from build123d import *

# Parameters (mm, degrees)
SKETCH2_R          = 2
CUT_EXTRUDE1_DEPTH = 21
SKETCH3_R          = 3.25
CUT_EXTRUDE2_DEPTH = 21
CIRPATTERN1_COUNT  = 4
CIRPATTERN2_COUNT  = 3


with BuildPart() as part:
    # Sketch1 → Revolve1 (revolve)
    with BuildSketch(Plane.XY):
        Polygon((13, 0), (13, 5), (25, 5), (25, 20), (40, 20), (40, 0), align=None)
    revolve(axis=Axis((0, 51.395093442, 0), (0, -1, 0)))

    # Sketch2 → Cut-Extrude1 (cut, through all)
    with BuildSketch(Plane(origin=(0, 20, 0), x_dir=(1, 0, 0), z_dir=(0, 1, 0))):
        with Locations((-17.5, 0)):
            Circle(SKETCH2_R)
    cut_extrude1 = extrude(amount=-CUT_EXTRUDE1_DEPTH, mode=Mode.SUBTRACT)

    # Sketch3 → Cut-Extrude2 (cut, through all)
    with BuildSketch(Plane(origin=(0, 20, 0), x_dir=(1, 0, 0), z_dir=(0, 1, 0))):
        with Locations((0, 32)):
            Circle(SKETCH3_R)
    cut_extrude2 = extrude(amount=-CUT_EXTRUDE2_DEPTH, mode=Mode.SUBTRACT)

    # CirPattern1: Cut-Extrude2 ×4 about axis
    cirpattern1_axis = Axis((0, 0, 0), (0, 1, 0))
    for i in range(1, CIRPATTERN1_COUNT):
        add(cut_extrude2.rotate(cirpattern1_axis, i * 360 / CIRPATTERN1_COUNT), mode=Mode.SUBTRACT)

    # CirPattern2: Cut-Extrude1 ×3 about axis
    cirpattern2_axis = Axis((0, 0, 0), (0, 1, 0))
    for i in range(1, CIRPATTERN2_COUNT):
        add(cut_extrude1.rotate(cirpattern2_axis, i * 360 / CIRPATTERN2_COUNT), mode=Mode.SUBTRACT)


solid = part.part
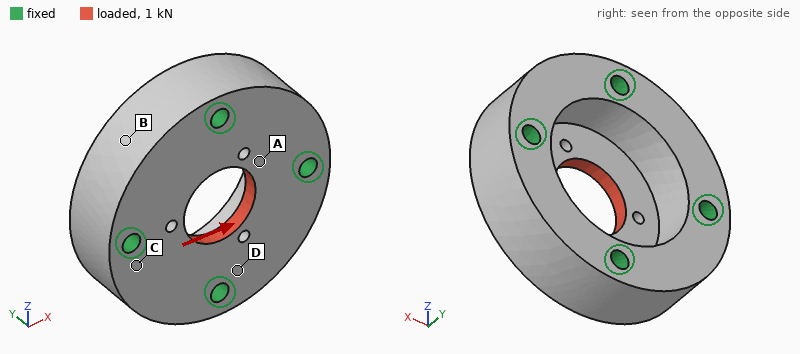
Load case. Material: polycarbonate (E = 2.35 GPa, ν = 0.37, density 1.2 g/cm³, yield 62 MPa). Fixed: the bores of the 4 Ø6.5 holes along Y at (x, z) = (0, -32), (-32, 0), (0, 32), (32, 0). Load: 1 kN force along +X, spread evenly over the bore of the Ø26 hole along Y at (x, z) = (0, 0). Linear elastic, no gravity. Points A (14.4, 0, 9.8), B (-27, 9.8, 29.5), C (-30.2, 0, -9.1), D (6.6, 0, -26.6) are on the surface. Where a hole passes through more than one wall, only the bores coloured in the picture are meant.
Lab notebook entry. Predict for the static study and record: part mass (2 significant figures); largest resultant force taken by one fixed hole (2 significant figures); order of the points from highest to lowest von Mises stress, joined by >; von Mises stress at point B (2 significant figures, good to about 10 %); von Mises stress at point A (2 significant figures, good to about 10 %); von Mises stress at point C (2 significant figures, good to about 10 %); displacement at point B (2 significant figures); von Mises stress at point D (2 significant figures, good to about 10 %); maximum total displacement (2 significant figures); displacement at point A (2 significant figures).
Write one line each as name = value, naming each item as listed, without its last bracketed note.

part mass = 79 g
largest resultant force taken by one fixed hole = 280 N
order of the points from highest to lowest von Mises stress, joined by > = A > C > D > B
von Mises stress at point B = 0.49 MPa
von Mises stress at point A = 2.4 MPa
von Mises stress at point C = 1.5 MPa
displacement at point B = 8.4 µm
von Mises stress at point D = 1.0 MPa
maximum total displacement = 33 µm
displacement at point A = 22 µm
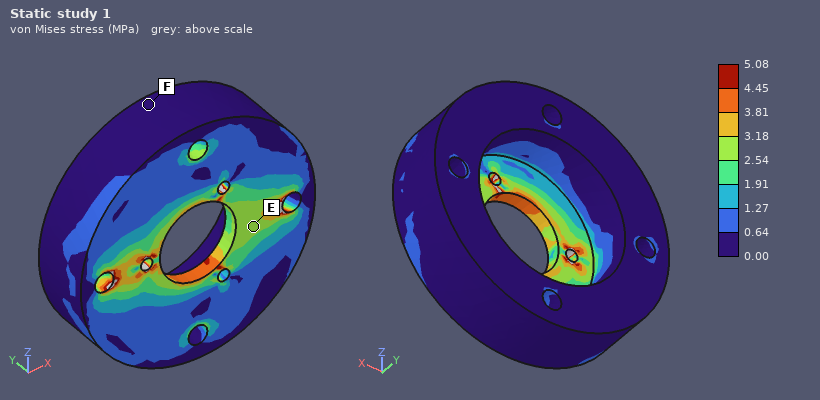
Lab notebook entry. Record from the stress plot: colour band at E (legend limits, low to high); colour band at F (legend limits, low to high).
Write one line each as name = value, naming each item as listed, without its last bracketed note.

colour band at E = 2.54 to 3.18 MPa
colour band at F = 0.00 to 0.64 MPa
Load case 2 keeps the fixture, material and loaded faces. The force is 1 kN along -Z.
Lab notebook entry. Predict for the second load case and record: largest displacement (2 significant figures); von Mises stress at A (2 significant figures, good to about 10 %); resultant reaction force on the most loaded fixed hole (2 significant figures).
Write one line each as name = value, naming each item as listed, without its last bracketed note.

largest displacement = 33 µm
von Mises stress at A = 1.8 MPa
resultant reaction force on the most loaded fixed hole = 280 N
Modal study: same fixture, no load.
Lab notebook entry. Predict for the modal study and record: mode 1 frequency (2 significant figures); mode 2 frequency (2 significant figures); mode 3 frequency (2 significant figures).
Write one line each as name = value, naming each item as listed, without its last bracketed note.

mode 1 frequency = 6100 Hz
mode 2 frequency = 6100 Hz
mode 3 frequency = 6300 Hz
